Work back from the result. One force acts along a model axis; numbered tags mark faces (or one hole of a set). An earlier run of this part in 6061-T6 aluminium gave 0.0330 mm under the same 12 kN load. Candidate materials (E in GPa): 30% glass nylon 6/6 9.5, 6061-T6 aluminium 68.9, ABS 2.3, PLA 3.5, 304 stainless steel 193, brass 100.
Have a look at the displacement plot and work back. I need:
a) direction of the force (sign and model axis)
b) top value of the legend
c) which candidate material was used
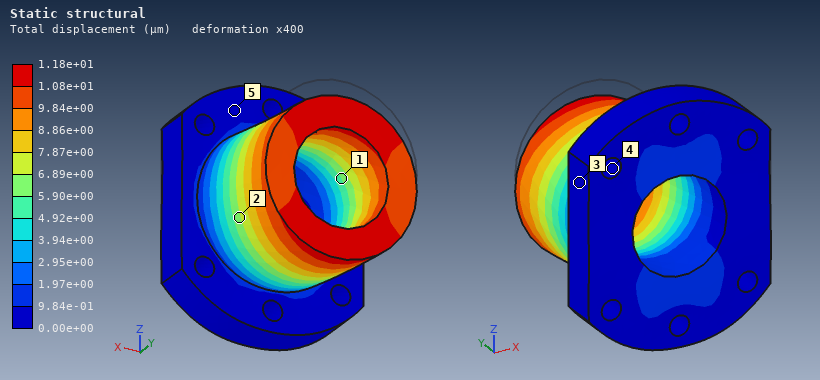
-Z
1.18e+01 µm
304 stainless steel
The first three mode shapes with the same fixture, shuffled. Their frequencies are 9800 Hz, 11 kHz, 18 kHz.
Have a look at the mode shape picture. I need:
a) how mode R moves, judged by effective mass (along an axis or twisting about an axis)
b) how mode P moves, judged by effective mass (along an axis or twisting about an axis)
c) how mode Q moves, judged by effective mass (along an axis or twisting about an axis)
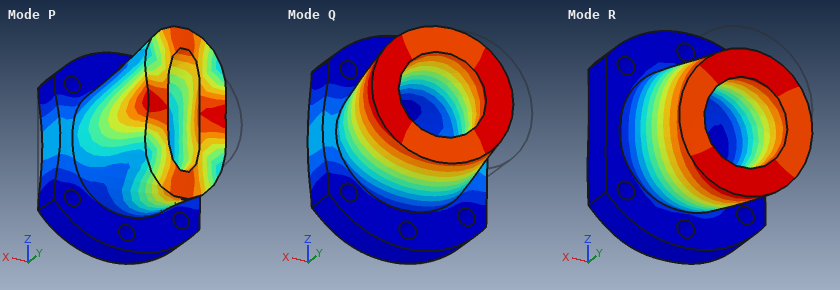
along Z
along Y
along X
